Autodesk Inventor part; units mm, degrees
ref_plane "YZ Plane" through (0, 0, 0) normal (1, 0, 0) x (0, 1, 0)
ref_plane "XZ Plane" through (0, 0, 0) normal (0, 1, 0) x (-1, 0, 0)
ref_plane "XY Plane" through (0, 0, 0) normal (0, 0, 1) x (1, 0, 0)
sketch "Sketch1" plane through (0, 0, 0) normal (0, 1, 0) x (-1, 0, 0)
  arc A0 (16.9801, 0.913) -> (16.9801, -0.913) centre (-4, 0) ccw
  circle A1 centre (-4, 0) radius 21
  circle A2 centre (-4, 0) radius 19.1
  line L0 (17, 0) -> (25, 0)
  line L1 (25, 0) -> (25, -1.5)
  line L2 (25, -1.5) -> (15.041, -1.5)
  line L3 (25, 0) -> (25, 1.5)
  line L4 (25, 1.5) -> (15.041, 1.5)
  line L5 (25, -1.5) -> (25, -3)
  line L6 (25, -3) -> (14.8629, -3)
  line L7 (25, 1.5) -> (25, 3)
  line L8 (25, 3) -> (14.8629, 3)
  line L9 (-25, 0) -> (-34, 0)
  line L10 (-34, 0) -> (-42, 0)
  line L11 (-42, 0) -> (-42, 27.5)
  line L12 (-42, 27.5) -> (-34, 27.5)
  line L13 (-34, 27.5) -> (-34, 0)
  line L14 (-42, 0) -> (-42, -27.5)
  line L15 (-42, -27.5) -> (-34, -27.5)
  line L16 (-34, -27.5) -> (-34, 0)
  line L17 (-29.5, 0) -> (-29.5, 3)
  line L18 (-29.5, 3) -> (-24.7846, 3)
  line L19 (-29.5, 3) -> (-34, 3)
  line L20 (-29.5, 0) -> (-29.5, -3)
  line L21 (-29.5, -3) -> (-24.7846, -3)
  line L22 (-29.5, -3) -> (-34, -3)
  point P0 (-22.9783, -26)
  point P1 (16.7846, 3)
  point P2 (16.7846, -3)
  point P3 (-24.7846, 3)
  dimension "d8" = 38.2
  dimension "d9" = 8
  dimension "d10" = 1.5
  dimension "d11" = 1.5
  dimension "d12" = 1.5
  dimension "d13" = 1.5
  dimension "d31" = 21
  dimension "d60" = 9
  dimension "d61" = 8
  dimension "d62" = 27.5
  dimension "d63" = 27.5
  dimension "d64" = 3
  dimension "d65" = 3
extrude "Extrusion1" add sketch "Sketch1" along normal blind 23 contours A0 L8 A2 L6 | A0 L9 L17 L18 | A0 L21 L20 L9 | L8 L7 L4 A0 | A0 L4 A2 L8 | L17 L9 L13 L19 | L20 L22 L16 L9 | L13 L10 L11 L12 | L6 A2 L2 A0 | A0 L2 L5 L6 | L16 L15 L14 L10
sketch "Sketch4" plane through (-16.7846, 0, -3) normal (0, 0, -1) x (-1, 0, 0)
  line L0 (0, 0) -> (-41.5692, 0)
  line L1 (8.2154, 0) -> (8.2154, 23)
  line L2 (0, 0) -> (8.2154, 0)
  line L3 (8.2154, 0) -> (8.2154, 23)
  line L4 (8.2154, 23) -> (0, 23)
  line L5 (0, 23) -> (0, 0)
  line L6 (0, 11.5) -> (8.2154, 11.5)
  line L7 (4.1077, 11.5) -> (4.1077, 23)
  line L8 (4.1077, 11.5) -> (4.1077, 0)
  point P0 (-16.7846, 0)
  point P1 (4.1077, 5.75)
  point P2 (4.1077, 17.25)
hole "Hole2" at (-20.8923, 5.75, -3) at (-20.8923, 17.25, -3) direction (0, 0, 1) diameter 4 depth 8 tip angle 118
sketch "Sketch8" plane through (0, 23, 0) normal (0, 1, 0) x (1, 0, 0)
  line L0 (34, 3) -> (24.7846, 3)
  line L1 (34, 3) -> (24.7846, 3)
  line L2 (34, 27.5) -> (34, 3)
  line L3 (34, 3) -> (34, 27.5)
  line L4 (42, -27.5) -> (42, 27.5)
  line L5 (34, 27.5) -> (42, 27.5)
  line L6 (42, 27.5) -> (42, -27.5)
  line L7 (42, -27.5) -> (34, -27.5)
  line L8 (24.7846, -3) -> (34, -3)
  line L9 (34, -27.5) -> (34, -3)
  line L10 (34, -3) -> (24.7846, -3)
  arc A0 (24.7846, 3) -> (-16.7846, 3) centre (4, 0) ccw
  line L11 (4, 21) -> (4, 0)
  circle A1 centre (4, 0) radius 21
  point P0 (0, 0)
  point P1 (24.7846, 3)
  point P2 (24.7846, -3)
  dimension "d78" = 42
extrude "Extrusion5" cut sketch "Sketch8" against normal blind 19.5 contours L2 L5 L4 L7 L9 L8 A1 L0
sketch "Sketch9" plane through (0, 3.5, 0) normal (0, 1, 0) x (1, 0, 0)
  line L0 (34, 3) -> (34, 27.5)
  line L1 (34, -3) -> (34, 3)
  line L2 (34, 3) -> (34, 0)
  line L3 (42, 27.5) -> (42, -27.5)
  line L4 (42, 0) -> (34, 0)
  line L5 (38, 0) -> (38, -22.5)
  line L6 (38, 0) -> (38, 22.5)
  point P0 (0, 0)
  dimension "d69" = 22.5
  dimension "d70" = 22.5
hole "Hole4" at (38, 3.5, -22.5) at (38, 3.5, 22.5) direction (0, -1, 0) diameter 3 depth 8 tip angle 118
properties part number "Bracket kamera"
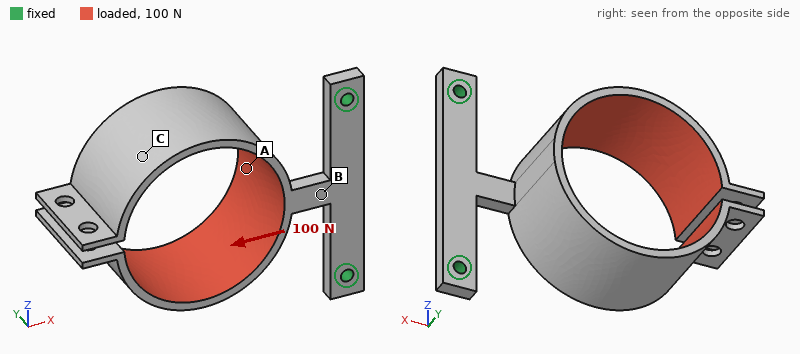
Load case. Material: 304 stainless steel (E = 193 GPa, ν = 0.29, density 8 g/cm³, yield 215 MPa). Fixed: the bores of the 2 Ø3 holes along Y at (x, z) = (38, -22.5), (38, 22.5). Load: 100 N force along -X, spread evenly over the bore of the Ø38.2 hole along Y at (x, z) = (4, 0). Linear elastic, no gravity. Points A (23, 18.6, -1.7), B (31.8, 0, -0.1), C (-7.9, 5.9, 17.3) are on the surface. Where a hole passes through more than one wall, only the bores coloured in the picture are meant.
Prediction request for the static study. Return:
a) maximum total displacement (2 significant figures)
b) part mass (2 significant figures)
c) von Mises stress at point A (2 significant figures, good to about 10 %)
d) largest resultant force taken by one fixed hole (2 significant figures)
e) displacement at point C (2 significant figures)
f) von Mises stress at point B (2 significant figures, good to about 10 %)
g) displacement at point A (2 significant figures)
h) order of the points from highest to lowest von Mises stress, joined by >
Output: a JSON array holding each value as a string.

["0.34 mm", "60 g", "31 MPa", "50 N", "0.22 mm", "73 MPa", "0.10 mm", "B > A > C"]
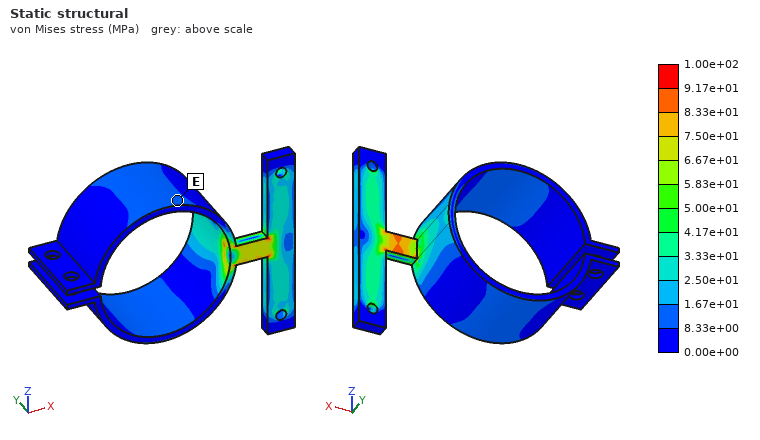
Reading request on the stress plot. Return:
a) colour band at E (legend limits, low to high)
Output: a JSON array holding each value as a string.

["8.33e+00 to 1.67e+01 MPa"]
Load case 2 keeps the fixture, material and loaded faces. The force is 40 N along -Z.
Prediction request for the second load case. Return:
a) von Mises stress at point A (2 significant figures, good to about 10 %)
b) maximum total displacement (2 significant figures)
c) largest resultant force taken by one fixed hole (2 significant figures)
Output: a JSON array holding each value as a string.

["18 MPa", "0.29 mm", "47 N"]
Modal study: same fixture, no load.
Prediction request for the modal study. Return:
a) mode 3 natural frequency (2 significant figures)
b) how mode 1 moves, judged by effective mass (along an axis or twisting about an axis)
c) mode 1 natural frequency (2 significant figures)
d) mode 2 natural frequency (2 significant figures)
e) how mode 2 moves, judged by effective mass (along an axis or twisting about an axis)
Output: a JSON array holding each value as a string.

["430 Hz", "along Y", "260 Hz", "310 Hz", "along Z"]
